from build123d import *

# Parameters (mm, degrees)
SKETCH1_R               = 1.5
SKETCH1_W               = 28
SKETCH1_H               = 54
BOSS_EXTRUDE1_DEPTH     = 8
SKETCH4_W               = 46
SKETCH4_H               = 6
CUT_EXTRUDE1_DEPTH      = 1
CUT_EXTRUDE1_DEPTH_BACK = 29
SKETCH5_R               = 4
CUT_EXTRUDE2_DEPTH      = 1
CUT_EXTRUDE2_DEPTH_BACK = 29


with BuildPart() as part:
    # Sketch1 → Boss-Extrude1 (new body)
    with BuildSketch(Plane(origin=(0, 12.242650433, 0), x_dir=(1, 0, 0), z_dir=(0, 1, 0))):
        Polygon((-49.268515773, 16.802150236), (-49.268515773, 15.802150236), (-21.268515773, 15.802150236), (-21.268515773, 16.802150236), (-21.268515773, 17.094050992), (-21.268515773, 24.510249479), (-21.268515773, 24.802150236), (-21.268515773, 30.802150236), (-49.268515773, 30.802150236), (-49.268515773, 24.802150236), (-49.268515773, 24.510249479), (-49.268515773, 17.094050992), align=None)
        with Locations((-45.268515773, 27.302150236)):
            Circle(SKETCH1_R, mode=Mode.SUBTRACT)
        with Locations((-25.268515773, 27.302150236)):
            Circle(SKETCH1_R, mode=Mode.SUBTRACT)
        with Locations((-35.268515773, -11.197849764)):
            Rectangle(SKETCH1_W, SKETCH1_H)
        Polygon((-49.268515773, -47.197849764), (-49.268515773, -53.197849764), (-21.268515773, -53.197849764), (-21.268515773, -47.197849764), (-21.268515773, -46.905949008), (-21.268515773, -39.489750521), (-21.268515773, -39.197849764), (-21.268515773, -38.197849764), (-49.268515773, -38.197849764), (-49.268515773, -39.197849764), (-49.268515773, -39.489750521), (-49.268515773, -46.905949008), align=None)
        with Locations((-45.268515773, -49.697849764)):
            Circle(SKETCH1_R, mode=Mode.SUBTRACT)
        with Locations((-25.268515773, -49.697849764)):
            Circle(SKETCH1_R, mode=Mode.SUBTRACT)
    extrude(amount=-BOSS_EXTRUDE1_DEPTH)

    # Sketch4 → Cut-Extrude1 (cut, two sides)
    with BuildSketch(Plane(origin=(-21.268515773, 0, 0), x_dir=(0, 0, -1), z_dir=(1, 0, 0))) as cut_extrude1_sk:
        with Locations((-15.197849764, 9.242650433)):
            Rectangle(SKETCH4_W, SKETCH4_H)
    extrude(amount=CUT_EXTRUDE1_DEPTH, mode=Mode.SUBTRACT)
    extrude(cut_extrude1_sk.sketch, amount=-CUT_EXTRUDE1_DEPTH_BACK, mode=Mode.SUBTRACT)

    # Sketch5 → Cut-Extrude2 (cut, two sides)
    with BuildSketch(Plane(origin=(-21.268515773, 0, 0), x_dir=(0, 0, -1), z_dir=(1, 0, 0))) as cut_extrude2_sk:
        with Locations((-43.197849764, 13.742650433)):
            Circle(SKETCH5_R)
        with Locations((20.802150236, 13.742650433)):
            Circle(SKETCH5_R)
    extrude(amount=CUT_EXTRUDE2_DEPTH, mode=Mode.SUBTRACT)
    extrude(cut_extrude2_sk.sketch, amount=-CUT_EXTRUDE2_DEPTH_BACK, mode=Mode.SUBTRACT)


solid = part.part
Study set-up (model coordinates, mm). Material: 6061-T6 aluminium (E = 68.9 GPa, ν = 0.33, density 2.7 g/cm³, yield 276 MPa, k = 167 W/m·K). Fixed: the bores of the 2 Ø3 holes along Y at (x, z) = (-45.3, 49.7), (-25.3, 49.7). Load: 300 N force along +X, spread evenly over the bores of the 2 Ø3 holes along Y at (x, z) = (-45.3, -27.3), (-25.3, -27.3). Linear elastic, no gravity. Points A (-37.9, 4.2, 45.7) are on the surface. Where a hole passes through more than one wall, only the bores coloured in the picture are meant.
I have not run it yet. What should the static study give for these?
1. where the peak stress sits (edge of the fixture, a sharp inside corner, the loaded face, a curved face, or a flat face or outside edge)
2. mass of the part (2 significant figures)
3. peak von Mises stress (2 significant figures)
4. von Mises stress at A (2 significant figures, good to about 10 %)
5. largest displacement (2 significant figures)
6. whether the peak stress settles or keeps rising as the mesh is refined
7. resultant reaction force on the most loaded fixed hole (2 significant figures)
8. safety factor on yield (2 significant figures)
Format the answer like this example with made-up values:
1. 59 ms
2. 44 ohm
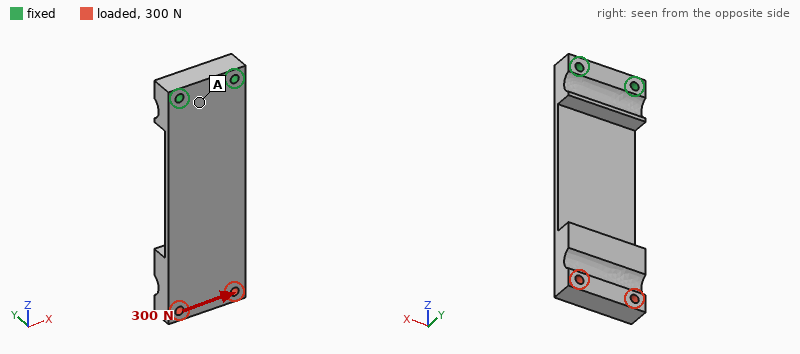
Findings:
1. a flat face or outside edge
2. 27 g
3. 110 MPa
4. 14 MPa
5. 0.40 mm
6. settles
7. 1.1 kN
8. 2.4
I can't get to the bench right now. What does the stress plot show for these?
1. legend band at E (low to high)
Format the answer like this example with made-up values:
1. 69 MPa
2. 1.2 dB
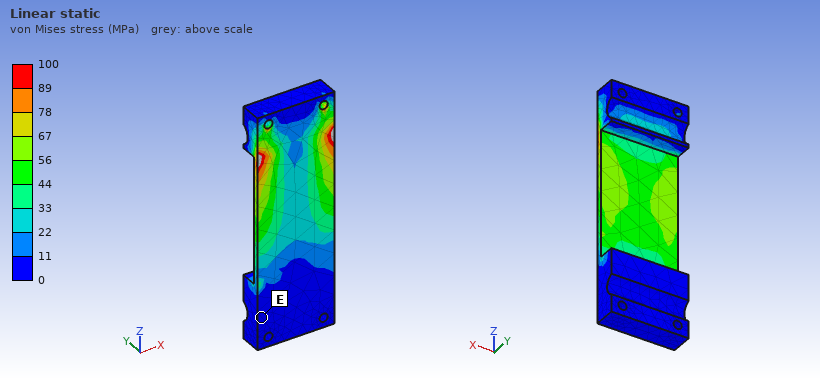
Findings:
1. 0 to 11 MPa
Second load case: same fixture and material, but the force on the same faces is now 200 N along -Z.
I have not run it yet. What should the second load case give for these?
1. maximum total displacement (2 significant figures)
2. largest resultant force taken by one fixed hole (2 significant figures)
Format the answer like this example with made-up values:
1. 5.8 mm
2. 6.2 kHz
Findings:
1. 0.99 mm
2. 100 N
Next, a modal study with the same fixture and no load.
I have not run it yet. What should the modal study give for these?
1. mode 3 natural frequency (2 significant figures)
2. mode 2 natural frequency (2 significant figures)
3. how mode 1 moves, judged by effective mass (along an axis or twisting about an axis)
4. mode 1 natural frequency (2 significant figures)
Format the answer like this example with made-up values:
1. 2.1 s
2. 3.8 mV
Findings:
1. 1700 Hz
2. 1100 Hz
3. along Y
4. 190 Hz
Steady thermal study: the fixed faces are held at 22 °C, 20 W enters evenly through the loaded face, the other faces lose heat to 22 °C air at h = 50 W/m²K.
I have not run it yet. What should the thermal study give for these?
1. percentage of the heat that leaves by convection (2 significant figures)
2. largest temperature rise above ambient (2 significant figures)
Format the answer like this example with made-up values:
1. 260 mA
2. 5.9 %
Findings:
1. 54 %
2. 71 K
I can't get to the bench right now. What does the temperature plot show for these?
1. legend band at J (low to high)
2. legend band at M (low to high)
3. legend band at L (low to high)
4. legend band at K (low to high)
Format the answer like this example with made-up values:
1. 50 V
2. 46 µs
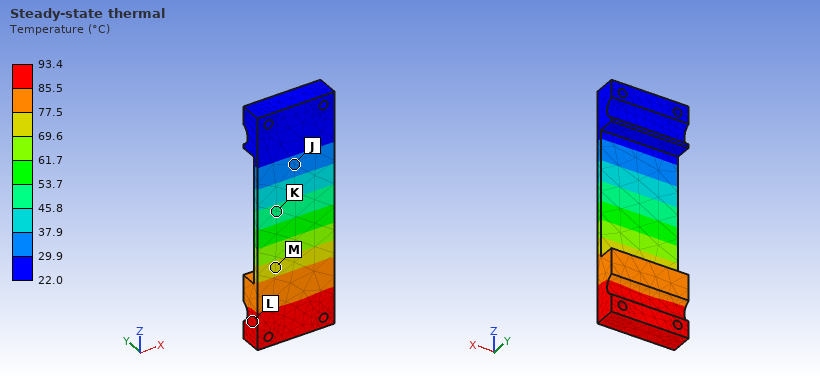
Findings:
1. 29.9 to 37.9 °C
2. 69.6 to 77.5 °C
3. 85.5 to 93.4 °C
4. 45.8 to 53.7 °C
